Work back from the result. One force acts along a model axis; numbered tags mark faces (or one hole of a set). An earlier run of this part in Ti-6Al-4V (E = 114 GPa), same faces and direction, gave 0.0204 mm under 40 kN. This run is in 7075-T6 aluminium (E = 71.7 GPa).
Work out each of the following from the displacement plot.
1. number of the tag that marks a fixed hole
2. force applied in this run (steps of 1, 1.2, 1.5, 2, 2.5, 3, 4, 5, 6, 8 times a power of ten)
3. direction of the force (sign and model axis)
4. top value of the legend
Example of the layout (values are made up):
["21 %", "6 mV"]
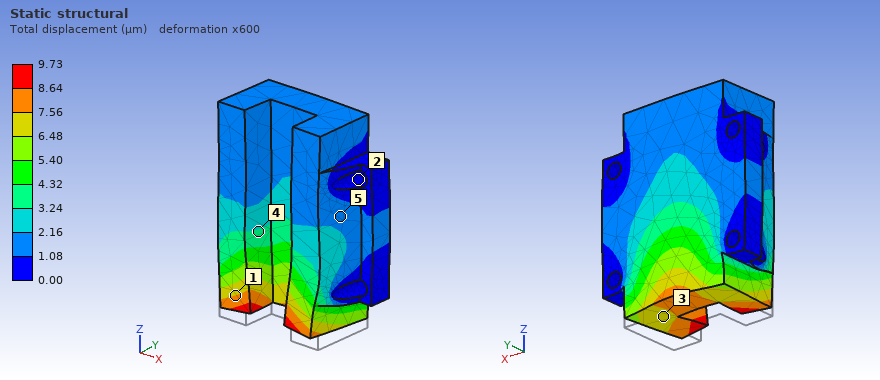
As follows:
["2", "12 kN", "+Z", "9.73 µm"]
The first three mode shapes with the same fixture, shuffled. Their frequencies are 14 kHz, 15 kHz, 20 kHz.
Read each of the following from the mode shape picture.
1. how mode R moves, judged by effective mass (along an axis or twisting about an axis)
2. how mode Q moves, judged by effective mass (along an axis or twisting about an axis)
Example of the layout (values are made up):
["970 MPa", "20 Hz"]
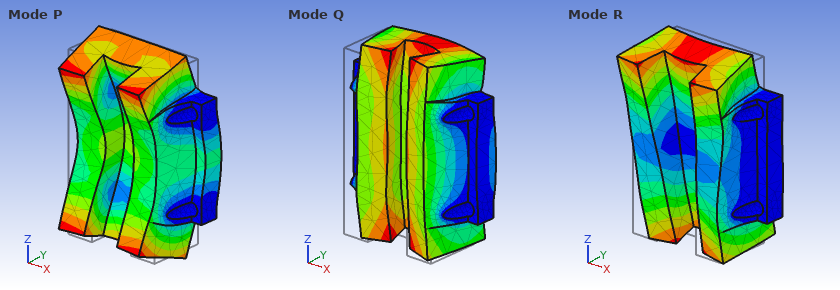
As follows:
["twisting about X", "along Y"]
